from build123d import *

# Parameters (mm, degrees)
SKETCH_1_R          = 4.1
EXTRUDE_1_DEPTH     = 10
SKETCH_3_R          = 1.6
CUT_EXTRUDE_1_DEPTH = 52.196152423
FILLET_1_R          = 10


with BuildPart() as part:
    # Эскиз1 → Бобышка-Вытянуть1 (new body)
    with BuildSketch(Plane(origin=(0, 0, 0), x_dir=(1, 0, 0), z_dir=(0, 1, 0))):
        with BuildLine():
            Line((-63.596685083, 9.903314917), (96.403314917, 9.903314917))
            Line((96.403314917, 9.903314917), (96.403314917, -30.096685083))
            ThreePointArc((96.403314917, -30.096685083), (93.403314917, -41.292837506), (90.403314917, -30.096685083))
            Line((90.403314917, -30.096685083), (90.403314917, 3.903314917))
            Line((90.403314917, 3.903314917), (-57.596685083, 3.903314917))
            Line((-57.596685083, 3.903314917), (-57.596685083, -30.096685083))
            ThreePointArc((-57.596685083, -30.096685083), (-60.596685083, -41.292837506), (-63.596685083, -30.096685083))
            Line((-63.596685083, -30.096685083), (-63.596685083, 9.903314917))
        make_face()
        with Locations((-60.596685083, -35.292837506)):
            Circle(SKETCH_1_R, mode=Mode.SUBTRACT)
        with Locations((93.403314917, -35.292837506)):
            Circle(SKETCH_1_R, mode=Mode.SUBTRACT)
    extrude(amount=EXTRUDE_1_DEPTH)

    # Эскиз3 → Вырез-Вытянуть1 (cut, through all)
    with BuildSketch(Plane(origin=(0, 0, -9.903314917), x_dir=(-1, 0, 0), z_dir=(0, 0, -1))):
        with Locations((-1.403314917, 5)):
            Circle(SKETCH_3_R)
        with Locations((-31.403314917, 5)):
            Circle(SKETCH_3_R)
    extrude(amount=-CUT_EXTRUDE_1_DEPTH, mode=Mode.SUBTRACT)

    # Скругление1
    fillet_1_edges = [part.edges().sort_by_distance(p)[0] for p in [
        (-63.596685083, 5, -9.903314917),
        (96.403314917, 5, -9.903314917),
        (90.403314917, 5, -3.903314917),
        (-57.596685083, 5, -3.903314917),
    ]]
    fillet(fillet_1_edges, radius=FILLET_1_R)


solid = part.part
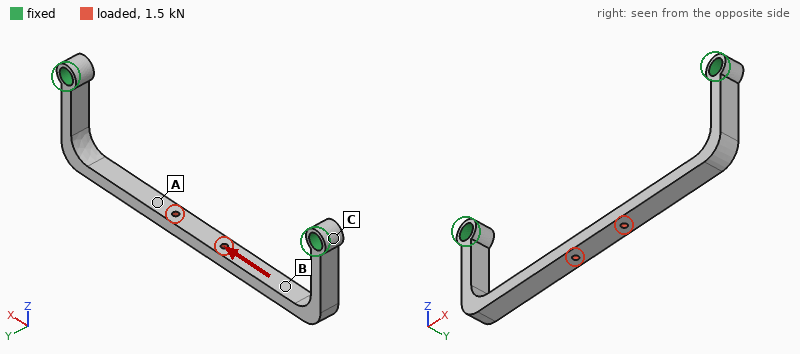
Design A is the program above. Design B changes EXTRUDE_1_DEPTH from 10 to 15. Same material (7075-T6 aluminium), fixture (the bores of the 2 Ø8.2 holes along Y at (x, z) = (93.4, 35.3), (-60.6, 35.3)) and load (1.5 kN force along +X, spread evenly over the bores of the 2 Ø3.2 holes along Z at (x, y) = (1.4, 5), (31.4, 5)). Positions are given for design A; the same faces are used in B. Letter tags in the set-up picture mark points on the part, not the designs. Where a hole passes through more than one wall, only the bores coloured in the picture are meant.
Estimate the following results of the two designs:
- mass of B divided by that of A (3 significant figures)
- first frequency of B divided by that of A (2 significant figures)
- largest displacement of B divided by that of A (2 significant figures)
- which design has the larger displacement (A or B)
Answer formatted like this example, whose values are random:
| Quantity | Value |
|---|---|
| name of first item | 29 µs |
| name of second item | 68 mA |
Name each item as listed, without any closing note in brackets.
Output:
| Quantity | Value |
|---|---|
| mass of B divided by that of A | 1.50 |
| first frequency of B divided by that of A | 1.2 |
| largest displacement of B divided by that of A | 0.66 |
| which design has the larger displacement | A |
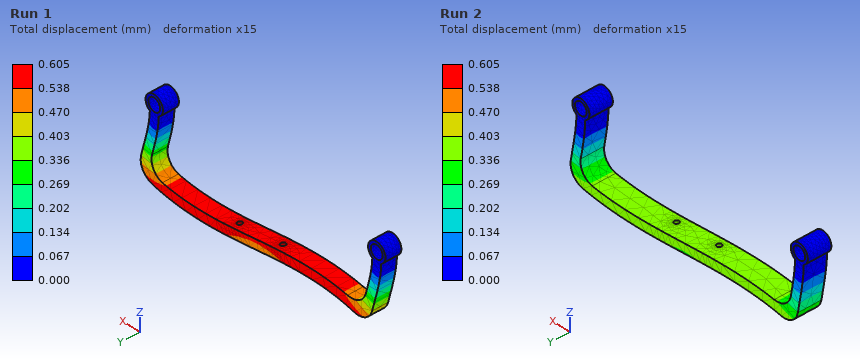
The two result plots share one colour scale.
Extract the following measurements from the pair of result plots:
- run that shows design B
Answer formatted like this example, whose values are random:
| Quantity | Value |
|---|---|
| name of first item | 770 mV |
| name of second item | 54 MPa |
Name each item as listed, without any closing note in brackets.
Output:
| Quantity | Value |
|---|---|
| run that shows design B | Run 2 |
